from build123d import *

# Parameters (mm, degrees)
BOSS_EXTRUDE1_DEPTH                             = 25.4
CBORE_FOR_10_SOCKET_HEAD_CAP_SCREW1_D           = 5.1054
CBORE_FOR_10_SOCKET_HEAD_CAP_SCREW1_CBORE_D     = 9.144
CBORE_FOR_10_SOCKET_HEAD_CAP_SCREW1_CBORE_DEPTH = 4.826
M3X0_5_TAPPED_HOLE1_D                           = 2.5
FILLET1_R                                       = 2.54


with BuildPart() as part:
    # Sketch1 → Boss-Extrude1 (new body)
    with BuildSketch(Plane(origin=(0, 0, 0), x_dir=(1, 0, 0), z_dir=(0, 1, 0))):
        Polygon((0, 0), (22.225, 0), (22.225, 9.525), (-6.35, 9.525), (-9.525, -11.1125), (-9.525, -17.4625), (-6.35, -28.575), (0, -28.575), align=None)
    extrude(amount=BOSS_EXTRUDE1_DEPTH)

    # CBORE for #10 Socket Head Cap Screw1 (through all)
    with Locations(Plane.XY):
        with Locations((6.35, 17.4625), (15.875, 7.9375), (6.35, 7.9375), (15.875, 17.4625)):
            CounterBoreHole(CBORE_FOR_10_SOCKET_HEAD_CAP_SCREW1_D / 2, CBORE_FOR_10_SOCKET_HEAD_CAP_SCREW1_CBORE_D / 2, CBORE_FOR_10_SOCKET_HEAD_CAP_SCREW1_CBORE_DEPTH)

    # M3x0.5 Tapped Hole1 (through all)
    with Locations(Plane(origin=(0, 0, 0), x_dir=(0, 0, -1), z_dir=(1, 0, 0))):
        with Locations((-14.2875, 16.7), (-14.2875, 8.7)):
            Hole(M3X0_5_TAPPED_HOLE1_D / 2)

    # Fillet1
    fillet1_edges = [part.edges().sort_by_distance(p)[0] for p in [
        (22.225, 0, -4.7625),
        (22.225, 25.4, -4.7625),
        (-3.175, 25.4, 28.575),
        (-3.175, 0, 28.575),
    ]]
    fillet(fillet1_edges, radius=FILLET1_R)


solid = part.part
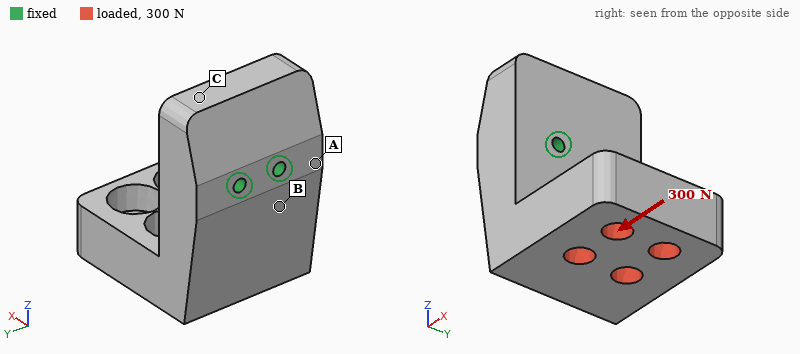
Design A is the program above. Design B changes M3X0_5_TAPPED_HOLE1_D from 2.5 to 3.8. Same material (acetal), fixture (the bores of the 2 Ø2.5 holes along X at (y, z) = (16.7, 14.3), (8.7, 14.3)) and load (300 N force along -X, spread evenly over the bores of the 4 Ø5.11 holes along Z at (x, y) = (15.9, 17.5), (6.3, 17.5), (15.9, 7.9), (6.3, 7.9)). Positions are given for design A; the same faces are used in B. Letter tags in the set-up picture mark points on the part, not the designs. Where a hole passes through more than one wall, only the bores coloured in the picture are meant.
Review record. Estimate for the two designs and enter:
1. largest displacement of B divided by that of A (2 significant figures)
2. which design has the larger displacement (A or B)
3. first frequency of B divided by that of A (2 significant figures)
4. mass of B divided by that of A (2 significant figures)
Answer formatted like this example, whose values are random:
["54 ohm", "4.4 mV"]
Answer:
["0.90", "A", "1.0", "0.99"]
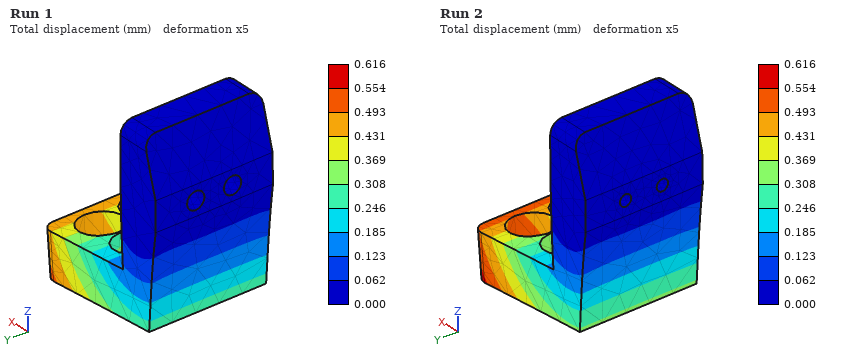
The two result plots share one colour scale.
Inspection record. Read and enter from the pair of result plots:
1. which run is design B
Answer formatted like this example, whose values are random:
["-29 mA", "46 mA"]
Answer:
["Run 1"]
